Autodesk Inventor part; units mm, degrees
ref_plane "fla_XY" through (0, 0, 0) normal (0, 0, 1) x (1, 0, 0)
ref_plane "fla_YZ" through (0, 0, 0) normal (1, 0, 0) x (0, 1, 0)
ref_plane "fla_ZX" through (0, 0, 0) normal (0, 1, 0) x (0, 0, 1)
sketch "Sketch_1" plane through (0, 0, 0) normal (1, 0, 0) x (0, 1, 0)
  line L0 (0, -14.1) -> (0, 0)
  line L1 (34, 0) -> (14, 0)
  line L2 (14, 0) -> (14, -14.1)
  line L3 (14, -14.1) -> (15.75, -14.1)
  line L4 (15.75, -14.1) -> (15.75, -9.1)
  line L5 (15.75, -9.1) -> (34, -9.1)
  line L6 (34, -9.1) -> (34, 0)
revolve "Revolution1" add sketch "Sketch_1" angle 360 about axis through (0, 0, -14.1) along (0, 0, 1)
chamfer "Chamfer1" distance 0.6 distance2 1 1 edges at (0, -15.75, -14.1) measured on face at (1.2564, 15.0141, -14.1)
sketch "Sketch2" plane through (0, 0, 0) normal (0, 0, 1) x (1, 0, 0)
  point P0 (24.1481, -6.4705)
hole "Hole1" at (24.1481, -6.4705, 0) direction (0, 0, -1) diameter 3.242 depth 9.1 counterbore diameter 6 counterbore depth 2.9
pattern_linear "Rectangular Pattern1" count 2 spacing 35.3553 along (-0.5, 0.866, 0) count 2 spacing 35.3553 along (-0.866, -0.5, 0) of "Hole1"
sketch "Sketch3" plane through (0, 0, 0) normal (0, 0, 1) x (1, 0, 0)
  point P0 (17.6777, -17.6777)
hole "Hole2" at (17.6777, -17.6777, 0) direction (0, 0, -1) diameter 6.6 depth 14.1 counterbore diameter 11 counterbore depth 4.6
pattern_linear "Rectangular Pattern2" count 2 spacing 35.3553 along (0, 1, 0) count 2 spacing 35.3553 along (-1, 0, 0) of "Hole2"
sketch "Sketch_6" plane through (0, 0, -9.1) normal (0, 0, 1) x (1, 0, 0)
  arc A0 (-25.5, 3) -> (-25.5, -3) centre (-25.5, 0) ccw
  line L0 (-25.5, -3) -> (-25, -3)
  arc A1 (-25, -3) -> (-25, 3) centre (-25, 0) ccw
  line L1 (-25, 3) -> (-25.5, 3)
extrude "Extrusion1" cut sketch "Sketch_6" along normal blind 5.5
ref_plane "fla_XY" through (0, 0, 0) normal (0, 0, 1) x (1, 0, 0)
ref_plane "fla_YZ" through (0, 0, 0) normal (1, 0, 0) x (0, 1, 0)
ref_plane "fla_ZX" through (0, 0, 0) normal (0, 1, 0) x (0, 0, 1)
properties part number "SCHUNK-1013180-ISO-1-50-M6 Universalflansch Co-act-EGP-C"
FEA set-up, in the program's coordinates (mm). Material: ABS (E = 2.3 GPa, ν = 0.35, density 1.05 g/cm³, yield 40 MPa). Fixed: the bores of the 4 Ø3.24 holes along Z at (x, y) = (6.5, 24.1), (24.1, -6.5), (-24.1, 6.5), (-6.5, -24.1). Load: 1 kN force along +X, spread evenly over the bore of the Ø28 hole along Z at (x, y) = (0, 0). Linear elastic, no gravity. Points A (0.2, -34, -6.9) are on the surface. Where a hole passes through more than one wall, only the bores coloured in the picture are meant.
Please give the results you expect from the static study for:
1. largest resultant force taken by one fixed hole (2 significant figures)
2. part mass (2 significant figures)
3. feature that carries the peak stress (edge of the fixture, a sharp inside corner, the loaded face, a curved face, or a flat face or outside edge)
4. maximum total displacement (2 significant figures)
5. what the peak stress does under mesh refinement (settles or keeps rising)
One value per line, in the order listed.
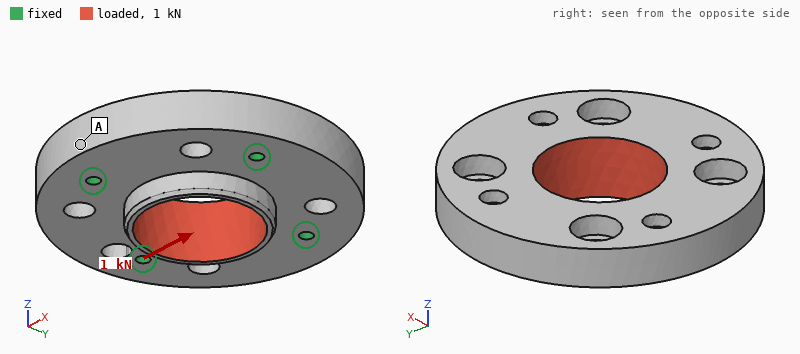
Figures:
260 N
26 g
edge of the fixture
75 µm
keeps rising
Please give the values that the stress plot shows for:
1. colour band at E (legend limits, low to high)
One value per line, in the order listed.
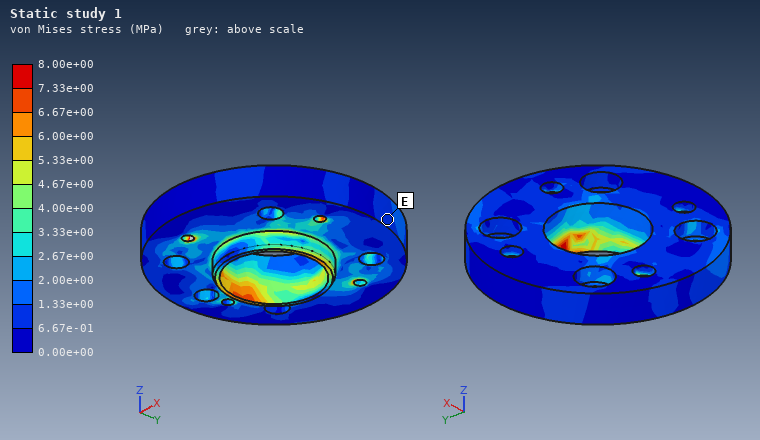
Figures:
6.67e-01 to 1.33e+00 MPa
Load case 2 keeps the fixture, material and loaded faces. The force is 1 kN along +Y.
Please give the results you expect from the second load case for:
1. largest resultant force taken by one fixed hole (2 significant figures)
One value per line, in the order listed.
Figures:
270 N
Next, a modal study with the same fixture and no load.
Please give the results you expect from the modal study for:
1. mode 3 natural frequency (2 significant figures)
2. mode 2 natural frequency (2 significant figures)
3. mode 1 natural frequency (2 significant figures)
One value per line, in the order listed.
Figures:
4500 Hz
4400 Hz
3600 Hz
